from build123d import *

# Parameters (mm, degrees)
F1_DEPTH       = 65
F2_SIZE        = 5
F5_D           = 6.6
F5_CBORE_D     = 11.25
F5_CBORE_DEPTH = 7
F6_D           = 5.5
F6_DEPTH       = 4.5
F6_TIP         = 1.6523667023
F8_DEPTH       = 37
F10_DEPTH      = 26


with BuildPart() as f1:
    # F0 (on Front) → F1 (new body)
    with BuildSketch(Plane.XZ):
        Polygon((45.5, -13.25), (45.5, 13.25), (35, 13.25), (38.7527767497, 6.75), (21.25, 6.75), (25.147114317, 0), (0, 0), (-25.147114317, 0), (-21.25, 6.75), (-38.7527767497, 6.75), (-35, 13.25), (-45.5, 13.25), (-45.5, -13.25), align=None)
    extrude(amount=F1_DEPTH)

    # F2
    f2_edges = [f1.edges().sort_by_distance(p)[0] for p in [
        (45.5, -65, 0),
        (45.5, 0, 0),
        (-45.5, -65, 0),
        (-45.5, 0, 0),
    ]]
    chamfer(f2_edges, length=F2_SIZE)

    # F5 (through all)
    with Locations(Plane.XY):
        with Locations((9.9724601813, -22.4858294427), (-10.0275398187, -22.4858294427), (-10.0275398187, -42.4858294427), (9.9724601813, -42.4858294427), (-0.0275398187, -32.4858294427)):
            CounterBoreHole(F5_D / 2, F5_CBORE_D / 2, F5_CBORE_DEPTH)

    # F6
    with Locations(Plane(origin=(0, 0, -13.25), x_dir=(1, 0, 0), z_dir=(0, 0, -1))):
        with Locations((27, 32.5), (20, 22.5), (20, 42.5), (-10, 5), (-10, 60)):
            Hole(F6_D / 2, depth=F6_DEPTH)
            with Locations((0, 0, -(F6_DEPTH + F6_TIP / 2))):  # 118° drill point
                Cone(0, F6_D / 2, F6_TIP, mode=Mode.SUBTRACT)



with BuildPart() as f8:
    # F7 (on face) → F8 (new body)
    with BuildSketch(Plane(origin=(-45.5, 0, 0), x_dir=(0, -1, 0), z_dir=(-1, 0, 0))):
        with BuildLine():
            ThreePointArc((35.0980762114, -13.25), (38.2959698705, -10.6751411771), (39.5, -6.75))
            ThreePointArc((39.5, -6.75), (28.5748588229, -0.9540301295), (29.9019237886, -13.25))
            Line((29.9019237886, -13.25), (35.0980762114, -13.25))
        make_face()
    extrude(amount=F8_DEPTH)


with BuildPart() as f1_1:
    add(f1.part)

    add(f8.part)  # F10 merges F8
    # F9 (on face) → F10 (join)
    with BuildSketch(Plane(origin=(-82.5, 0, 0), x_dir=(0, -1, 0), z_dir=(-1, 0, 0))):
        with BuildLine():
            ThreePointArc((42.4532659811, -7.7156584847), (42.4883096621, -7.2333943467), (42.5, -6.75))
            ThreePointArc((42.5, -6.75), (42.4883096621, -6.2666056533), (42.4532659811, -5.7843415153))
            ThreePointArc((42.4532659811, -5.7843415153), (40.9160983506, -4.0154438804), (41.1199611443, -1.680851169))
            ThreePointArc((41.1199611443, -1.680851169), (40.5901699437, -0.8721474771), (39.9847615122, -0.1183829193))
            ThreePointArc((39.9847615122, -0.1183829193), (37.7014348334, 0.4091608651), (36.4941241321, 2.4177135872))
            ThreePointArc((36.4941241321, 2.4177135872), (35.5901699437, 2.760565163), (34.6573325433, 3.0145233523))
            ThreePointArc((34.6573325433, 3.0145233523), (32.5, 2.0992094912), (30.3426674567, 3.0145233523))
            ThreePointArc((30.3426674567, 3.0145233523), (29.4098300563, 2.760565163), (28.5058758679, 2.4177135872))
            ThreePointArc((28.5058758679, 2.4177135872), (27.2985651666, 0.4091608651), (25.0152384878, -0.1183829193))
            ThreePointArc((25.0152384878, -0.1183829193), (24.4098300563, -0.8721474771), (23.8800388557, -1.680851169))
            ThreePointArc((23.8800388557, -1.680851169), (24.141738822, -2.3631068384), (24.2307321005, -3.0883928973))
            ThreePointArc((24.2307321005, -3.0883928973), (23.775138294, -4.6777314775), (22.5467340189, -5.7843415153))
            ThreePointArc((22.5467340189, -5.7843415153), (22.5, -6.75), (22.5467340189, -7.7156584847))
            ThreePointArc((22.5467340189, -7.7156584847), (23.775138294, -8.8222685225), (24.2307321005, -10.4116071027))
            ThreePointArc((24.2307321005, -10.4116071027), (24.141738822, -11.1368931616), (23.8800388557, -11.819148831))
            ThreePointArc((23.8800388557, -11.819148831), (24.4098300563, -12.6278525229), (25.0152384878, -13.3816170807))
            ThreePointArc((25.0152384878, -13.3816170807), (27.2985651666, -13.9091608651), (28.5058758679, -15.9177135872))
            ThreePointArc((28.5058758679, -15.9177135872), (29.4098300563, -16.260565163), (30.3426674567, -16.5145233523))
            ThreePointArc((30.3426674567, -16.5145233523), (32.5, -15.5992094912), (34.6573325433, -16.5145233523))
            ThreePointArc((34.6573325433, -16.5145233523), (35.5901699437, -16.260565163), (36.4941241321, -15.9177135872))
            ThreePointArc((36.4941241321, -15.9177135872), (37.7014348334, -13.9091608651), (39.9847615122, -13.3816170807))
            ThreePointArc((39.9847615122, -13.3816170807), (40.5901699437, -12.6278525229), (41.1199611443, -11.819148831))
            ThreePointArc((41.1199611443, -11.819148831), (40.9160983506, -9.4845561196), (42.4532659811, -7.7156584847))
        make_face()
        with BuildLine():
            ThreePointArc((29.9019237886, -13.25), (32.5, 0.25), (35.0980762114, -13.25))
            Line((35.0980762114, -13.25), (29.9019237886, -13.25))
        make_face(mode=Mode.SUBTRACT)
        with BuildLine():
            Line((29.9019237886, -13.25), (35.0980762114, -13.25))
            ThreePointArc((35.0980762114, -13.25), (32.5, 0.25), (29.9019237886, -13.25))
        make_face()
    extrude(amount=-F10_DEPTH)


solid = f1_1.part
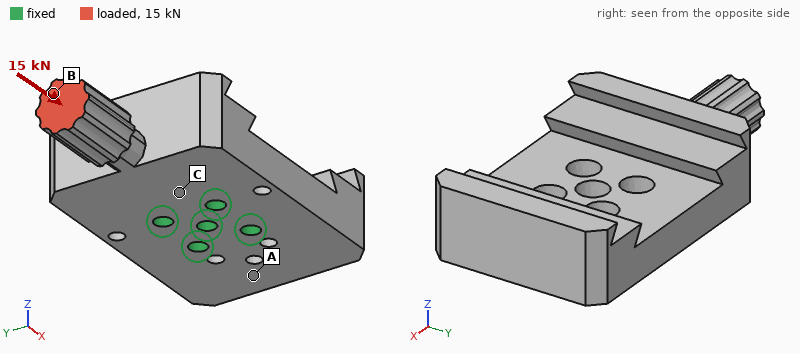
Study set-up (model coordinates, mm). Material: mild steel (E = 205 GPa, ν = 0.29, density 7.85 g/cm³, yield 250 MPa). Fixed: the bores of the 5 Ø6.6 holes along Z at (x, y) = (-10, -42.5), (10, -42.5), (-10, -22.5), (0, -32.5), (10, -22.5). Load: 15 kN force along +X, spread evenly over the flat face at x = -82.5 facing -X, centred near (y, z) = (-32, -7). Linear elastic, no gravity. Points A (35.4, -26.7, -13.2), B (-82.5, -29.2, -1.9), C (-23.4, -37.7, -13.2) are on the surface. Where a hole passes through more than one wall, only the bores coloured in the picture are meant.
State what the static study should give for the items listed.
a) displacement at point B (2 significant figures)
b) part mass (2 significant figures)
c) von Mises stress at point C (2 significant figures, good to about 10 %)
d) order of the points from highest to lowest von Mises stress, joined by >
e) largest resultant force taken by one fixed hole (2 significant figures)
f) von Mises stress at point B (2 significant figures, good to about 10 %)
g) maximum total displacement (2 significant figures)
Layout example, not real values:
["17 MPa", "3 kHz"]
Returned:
["21 µm", "850 g", "41 MPa", "B > C > A", "5.4 kN", "53 MPa", "22 µm"]
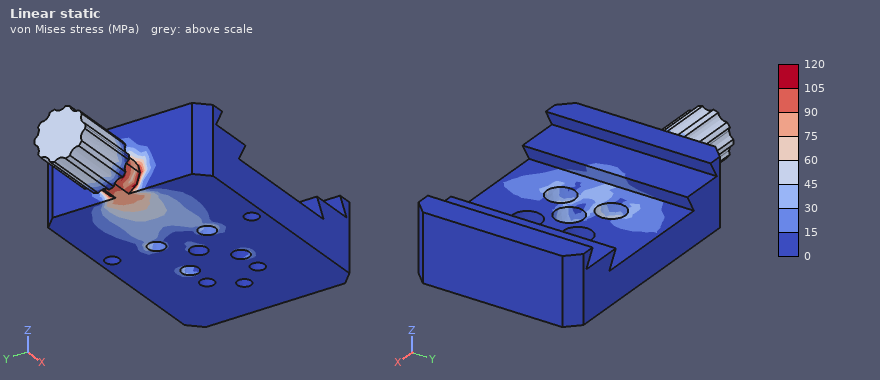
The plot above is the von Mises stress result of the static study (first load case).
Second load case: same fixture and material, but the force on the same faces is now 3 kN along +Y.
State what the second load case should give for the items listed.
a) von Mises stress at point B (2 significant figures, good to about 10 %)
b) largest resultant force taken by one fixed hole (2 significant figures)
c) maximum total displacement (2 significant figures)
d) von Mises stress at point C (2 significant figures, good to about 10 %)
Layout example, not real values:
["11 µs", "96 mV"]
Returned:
["20 MPa", "5.1 kN", "0.18 mm", "21 MPa"]
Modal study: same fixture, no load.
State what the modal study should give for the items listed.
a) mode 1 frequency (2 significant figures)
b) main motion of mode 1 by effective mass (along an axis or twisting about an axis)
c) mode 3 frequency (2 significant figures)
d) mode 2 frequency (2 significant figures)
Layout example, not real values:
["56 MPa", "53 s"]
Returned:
["2300 Hz", "along Z", "4100 Hz", "3900 Hz"]
